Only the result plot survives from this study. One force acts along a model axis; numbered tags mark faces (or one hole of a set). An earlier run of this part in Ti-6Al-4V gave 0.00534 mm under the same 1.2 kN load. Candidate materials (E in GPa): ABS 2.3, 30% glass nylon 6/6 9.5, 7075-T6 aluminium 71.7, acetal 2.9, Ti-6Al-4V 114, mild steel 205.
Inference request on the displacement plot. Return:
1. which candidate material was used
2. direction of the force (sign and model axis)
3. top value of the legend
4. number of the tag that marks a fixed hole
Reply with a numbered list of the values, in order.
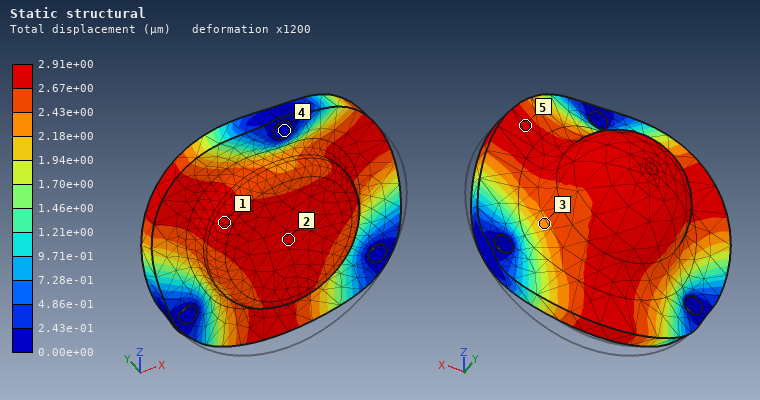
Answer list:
1. mild steel
2. +Y
3. 2.91e+00 µm
4. 4
